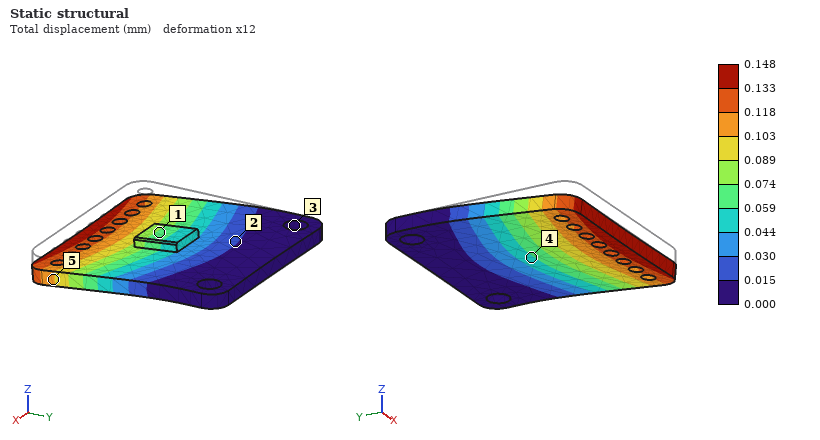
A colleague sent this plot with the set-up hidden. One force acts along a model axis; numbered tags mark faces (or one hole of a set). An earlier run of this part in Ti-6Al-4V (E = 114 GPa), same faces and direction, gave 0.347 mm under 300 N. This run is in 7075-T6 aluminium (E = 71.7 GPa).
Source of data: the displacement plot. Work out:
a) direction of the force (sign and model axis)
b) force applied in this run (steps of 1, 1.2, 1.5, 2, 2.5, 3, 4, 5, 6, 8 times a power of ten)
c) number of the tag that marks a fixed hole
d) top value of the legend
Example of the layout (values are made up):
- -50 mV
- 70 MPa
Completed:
- -Z
- 80 N
- 3
- 0.148 mm
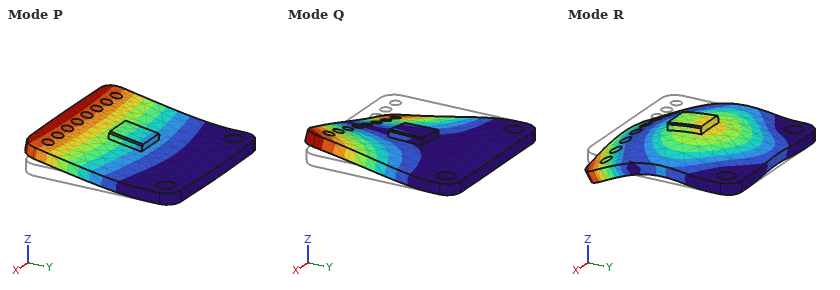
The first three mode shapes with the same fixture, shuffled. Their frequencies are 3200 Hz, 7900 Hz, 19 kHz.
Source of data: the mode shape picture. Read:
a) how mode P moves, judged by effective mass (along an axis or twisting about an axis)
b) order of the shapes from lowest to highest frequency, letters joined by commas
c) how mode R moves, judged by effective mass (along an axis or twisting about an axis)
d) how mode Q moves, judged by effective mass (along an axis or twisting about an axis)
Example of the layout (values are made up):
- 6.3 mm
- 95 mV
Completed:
- along Z
- P, Q, R
- along Z
- twisting about Y
